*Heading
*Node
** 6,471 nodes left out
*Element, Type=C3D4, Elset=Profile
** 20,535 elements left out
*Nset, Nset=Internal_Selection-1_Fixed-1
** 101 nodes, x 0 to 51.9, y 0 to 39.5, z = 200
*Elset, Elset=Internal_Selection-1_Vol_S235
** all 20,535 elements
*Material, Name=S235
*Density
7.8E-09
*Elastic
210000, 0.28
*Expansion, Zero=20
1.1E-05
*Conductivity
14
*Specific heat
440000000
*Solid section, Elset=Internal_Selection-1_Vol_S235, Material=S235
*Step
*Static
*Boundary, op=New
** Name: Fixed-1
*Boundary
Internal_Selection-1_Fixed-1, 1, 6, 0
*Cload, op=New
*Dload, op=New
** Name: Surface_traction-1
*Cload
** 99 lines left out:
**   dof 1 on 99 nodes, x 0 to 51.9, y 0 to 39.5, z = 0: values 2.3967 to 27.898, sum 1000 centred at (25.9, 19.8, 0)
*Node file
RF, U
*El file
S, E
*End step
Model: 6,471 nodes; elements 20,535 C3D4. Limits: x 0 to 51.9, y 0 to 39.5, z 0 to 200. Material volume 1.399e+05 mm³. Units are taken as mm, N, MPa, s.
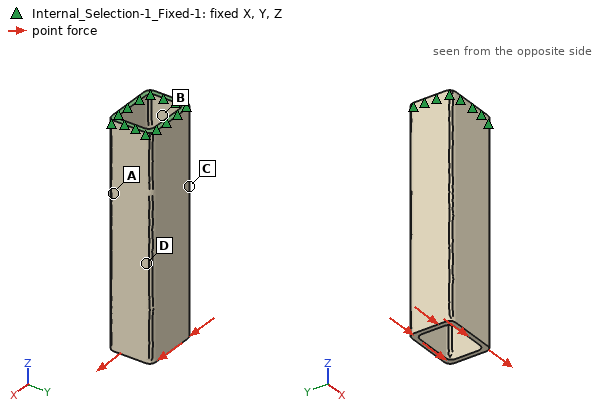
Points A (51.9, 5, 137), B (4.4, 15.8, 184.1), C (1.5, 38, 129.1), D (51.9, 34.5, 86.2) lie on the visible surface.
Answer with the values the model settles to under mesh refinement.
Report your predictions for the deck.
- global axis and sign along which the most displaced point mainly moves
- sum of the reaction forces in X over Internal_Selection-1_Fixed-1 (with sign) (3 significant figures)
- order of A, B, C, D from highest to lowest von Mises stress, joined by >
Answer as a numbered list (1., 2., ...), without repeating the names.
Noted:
1. +X
2. -1000 N
3. B > A > C > D
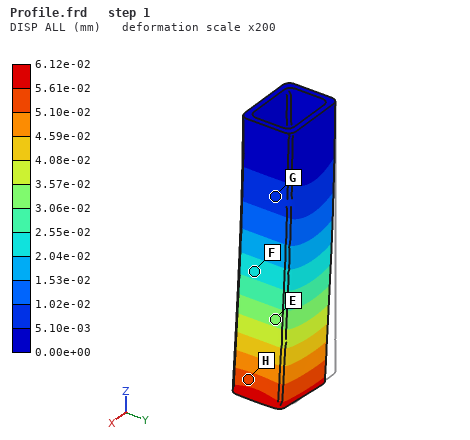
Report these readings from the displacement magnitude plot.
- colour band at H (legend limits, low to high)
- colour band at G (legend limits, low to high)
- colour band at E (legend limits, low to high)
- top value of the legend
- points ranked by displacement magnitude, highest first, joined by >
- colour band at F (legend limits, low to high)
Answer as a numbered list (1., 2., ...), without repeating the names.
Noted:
1. 5.10e-02 to 5.61e-02 mm
2. 5.10e-03 to 1.02e-02 mm
3. 3.06e-02 to 3.57e-02 mm
4. 6.12e-02 mm
5. H > E > F > G
6. 2.04e-02 to 2.55e-02 mm
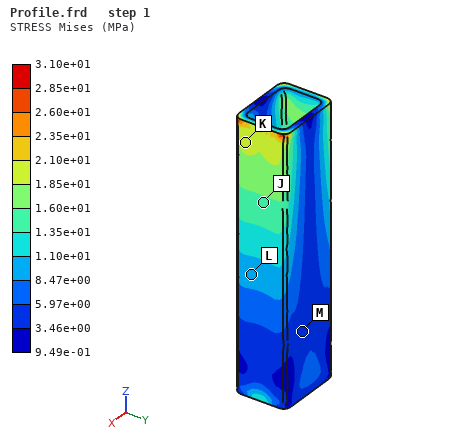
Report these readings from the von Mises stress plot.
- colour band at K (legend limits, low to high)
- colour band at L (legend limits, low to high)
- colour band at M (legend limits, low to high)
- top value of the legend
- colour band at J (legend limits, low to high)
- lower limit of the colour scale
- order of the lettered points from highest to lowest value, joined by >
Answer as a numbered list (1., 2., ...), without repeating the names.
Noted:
1. 1.85e+01 to 2.10e+01 MPa
2. 8.47e+00 to 1.10e+01 MPa
3. 3.46e+00 to 5.97e+00 MPa
4. 3.10e+01 MPa
5. 1.35e+01 to 1.60e+01 MPa
6. 9.49e-01 MPa
7. K > J > L > M
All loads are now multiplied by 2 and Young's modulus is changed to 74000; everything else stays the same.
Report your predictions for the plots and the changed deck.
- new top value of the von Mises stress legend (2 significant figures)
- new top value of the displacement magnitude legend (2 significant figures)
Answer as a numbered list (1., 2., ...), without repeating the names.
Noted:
1. 62 MPa
2. 0.35 mm
